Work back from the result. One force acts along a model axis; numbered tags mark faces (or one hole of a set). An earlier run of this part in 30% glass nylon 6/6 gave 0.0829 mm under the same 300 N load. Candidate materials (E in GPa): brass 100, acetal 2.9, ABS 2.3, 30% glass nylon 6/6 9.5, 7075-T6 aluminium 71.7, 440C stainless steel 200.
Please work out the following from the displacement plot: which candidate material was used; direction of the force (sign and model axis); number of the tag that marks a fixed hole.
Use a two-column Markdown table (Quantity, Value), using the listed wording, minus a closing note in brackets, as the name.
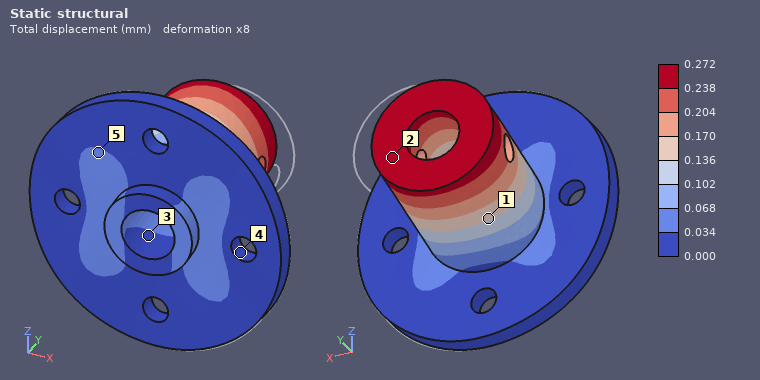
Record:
| Quantity | Value |
|---|---|
| which candidate material was used | acetal |
| direction of the force | -X |
| number of the tag that marks a fixed hole | 4 |
